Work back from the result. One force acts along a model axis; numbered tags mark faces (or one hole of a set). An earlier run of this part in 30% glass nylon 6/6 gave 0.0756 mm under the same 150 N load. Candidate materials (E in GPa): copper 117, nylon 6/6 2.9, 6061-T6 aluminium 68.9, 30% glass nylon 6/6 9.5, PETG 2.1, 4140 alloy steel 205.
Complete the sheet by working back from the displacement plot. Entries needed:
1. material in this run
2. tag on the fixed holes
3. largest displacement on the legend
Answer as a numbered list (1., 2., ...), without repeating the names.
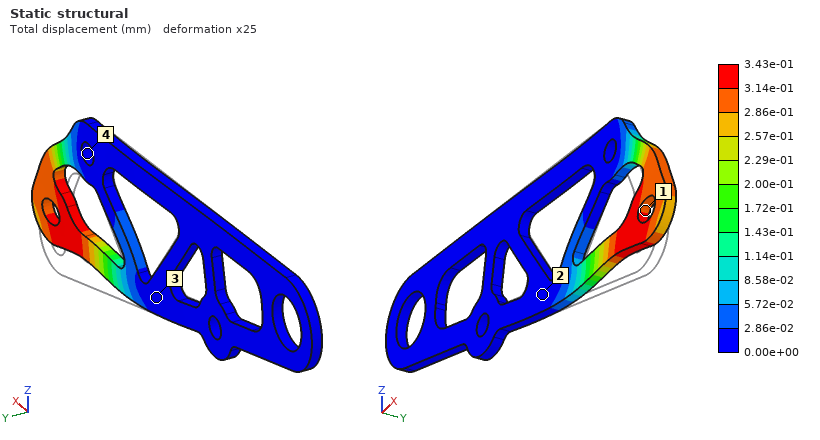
1. PETG
2. 4
3. 3.43e-01 mm
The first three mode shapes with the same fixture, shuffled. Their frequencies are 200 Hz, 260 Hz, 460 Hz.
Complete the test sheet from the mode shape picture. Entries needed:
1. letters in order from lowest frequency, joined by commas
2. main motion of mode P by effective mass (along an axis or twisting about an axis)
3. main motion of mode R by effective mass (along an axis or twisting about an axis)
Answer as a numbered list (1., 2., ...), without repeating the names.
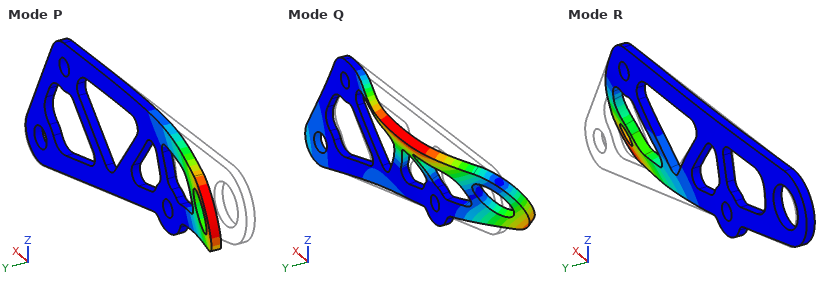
1. P, R, Q
2. along Y
3. along Y
